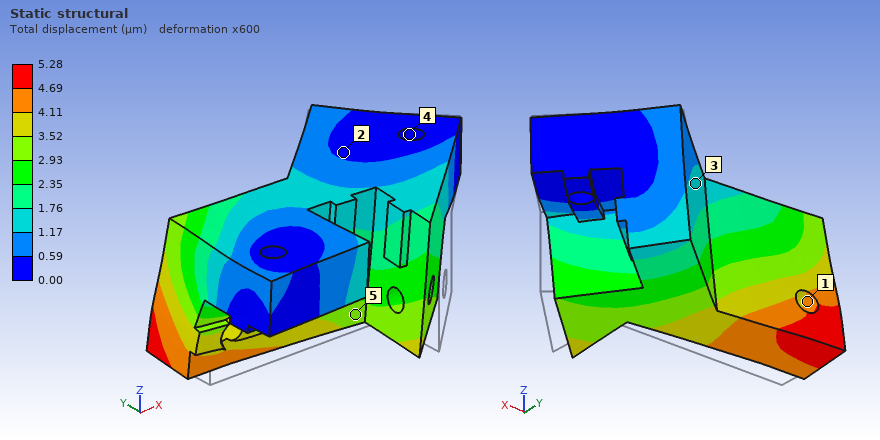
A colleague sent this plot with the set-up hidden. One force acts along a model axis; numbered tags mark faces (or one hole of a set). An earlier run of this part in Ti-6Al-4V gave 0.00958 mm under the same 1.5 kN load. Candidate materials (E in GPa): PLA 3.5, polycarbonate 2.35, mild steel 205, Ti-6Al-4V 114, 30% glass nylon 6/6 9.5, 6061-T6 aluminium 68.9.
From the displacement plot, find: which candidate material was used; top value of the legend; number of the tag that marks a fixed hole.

mild steel
5.28 µm
4
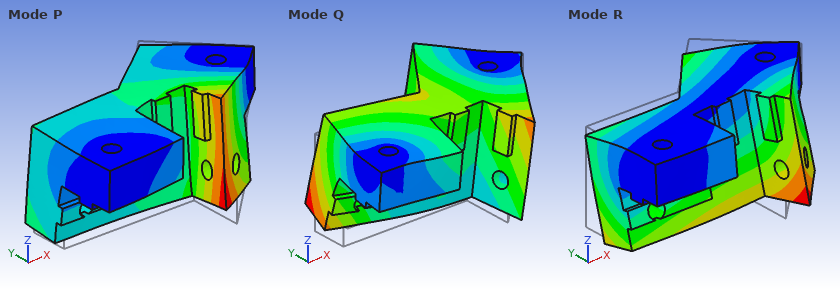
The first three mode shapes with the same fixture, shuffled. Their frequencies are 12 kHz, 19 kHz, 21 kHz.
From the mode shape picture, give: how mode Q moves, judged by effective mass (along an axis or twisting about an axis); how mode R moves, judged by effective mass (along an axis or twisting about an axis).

along Z
along Y
